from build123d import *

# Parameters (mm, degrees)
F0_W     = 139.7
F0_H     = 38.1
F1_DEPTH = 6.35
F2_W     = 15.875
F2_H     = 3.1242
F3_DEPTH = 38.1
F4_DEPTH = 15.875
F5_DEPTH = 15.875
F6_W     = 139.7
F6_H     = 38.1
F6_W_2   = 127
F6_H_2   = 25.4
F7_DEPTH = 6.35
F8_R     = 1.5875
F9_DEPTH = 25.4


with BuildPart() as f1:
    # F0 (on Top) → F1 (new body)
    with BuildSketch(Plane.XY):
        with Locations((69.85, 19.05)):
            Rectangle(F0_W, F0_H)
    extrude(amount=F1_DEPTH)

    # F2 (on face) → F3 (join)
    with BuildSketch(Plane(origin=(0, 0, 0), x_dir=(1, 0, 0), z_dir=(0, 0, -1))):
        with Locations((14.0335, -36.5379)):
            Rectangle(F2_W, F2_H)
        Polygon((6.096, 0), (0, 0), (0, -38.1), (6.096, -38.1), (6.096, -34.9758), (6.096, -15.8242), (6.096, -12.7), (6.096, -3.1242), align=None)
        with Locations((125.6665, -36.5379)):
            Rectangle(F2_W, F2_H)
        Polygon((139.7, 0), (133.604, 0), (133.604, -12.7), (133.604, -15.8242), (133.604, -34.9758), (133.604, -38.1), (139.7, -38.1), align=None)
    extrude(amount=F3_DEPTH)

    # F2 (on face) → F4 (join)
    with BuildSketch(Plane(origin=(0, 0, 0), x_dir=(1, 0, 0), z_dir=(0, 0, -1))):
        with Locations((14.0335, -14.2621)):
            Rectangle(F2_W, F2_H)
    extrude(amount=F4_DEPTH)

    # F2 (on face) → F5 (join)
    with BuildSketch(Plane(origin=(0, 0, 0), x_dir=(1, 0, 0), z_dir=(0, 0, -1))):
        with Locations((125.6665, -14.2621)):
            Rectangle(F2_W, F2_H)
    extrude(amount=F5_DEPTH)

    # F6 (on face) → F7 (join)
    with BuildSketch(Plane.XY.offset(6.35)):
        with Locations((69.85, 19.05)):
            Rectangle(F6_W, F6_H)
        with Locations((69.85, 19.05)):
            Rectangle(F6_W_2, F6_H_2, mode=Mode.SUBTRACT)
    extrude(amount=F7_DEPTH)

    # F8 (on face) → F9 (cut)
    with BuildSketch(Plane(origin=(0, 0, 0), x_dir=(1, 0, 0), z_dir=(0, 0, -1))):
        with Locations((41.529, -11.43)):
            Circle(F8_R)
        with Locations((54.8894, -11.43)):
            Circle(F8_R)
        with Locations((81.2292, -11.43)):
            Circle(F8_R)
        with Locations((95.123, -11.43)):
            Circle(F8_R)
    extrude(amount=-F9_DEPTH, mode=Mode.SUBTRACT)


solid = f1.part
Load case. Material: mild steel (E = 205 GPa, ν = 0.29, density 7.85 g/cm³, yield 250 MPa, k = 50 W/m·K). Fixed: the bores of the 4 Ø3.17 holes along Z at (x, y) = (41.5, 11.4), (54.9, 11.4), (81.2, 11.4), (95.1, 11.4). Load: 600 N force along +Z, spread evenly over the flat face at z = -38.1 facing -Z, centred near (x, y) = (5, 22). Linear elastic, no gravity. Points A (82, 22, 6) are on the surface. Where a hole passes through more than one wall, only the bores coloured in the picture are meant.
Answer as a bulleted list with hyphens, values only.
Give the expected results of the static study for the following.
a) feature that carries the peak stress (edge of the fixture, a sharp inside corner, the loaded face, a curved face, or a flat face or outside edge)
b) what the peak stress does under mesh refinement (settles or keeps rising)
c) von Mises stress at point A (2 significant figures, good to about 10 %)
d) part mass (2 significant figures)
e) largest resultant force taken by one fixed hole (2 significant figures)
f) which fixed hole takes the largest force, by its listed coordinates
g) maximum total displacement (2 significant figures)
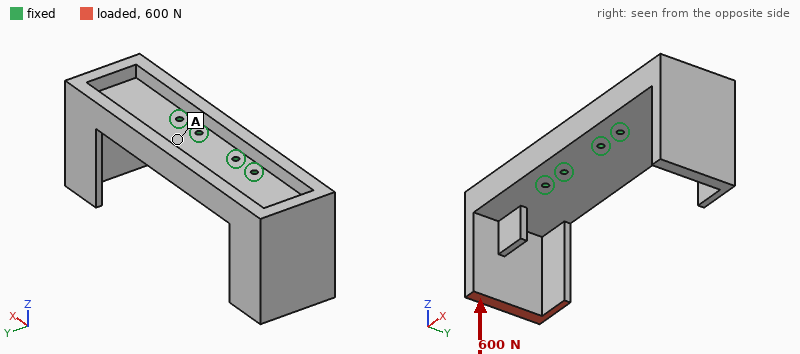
- edge of the fixture
- keeps rising
- 4.6 MPa
- 550 g
- 1.3 kN
- (41.5, 11.4)
- 67 µm
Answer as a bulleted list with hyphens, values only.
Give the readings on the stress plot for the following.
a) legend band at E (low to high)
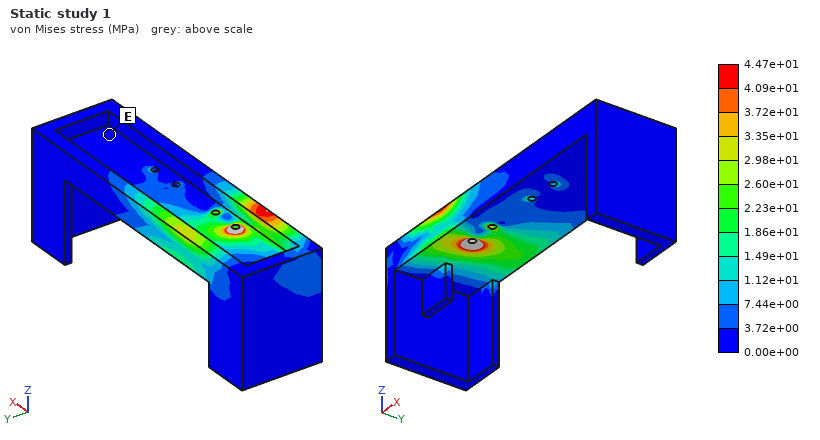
- 0.00e+00 to 3.72e+00 MPa
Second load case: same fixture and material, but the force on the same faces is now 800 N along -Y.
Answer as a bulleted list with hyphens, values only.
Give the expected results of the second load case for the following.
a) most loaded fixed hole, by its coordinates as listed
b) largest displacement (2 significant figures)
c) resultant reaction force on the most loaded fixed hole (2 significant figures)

- (41.5, 11.4)
- 0.19 mm
- 1.2 kN
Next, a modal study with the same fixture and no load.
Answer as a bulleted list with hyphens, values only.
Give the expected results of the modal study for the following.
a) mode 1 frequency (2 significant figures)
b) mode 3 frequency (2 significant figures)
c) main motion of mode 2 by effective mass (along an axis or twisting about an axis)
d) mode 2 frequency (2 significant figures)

- 1300 Hz
- 1900 Hz
- along Z
- 1500 Hz
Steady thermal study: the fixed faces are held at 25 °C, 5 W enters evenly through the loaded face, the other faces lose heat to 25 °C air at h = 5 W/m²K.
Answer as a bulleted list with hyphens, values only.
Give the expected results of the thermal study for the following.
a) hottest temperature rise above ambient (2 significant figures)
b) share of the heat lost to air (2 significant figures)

- 24 K
- 14 %
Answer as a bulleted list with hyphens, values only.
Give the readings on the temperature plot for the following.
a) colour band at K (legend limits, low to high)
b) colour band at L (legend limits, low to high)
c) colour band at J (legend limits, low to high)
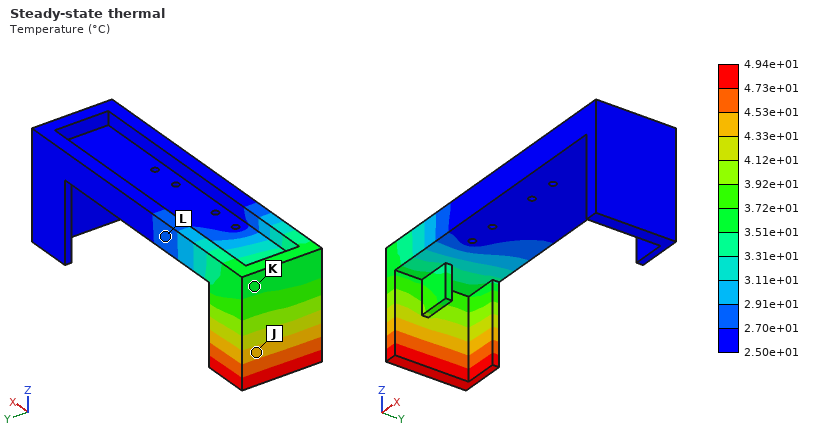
- 3.51e+01 to 3.72e+01 °C
- 2.70e+01 to 2.91e+01 °C
- 4.33e+01 to 4.53e+01 °C
